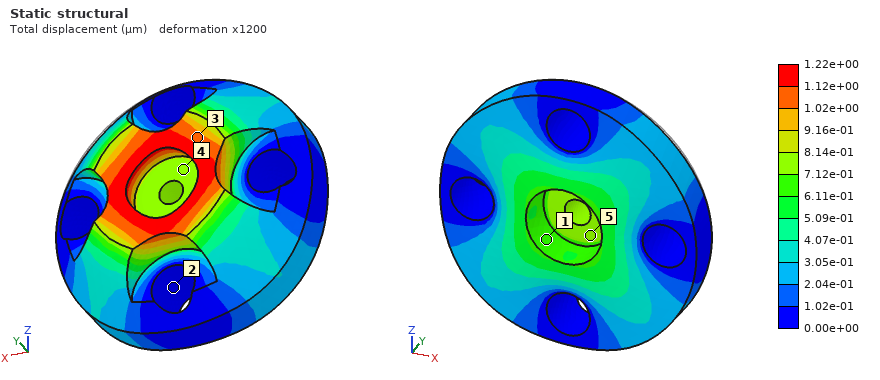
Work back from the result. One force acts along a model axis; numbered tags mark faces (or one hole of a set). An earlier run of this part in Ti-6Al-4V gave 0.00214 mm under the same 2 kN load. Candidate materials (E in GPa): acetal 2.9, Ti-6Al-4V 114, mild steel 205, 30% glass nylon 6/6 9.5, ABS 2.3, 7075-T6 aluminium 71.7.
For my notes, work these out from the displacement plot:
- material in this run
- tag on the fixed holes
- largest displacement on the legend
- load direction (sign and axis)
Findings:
mild steel
2
1.22e+00 µm
-Y
